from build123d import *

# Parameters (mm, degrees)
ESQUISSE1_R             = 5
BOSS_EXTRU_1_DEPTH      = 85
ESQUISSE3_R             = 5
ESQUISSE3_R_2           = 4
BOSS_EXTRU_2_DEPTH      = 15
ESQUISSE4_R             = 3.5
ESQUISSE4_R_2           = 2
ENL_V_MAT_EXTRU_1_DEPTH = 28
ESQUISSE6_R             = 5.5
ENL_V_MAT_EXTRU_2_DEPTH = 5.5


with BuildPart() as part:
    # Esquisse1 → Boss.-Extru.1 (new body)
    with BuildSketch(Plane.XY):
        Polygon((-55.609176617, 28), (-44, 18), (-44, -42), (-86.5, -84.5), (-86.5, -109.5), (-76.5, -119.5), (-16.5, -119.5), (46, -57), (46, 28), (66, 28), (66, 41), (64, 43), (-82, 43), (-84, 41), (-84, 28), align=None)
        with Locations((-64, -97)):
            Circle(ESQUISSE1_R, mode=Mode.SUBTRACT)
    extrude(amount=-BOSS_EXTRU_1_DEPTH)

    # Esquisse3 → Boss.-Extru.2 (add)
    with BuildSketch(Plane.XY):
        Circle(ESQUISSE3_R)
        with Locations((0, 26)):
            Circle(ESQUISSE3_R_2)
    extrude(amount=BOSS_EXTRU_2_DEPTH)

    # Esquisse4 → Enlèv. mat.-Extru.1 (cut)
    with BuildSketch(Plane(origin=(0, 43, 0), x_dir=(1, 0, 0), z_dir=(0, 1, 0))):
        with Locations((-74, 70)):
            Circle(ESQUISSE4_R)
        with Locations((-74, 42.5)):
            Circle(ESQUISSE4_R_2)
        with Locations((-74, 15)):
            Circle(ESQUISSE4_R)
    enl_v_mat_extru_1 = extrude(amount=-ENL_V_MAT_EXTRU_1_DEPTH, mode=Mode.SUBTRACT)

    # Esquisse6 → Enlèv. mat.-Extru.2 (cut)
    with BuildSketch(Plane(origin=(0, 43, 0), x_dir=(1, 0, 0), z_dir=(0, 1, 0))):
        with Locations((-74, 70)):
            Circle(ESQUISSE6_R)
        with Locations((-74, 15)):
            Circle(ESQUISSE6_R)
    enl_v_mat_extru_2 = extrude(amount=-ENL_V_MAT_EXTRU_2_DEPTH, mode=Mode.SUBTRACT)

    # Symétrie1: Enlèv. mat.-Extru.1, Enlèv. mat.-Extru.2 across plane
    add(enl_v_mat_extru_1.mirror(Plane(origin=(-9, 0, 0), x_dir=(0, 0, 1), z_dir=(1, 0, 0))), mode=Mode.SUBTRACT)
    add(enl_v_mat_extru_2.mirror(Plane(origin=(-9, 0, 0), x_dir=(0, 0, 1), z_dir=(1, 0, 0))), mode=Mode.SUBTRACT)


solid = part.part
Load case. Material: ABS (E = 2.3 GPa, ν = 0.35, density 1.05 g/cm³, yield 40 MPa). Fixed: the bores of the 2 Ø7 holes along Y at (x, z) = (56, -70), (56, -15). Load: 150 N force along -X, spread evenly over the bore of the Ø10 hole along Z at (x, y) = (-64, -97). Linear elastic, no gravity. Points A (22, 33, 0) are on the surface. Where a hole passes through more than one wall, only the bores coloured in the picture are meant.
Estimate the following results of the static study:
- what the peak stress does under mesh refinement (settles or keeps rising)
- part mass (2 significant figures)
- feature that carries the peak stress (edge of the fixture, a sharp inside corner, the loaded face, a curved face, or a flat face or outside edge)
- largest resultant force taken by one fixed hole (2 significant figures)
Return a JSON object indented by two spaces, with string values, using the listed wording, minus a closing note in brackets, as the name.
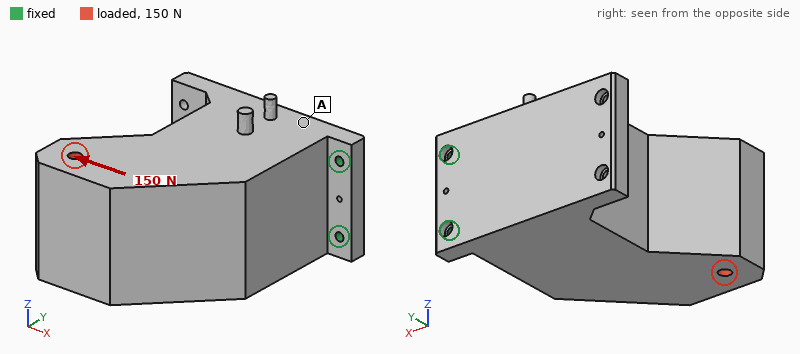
{
  "what the peak stress does under mesh refinement": "keeps rising",
  "part mass": "1.4 kg",
  "feature that carries the peak stress": "edge of the fixture",
  "largest resultant force taken by one fixed hole": "76 N"
}
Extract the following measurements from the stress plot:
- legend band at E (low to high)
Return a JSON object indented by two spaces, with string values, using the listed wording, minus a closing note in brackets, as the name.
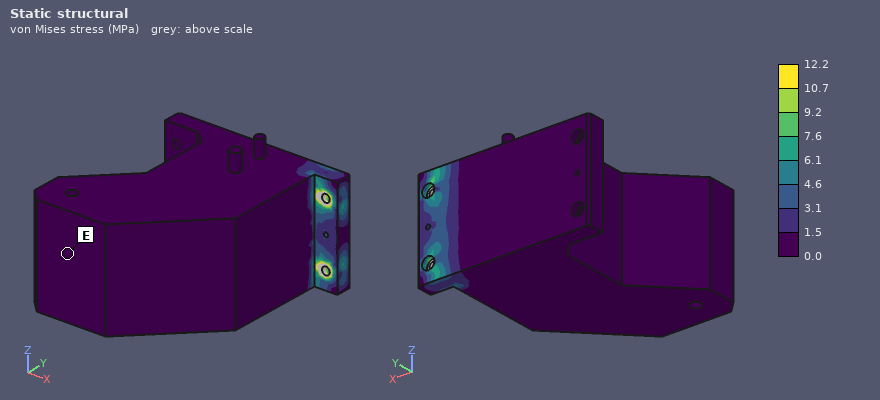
{
  "legend band at E": "0.0 to 1.5 MPa"
}
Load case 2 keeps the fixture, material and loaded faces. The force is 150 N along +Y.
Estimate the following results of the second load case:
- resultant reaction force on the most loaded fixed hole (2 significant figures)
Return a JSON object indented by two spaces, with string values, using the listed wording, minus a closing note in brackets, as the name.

{
  "resultant reaction force on the most loaded fixed hole": "76 N"
}
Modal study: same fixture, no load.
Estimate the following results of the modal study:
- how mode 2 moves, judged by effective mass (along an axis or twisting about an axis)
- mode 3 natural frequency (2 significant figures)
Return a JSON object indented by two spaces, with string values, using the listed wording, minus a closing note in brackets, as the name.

{
  "how mode 2 moves, judged by effective mass": "along Z",
  "mode 3 natural frequency": "500 Hz"
}
